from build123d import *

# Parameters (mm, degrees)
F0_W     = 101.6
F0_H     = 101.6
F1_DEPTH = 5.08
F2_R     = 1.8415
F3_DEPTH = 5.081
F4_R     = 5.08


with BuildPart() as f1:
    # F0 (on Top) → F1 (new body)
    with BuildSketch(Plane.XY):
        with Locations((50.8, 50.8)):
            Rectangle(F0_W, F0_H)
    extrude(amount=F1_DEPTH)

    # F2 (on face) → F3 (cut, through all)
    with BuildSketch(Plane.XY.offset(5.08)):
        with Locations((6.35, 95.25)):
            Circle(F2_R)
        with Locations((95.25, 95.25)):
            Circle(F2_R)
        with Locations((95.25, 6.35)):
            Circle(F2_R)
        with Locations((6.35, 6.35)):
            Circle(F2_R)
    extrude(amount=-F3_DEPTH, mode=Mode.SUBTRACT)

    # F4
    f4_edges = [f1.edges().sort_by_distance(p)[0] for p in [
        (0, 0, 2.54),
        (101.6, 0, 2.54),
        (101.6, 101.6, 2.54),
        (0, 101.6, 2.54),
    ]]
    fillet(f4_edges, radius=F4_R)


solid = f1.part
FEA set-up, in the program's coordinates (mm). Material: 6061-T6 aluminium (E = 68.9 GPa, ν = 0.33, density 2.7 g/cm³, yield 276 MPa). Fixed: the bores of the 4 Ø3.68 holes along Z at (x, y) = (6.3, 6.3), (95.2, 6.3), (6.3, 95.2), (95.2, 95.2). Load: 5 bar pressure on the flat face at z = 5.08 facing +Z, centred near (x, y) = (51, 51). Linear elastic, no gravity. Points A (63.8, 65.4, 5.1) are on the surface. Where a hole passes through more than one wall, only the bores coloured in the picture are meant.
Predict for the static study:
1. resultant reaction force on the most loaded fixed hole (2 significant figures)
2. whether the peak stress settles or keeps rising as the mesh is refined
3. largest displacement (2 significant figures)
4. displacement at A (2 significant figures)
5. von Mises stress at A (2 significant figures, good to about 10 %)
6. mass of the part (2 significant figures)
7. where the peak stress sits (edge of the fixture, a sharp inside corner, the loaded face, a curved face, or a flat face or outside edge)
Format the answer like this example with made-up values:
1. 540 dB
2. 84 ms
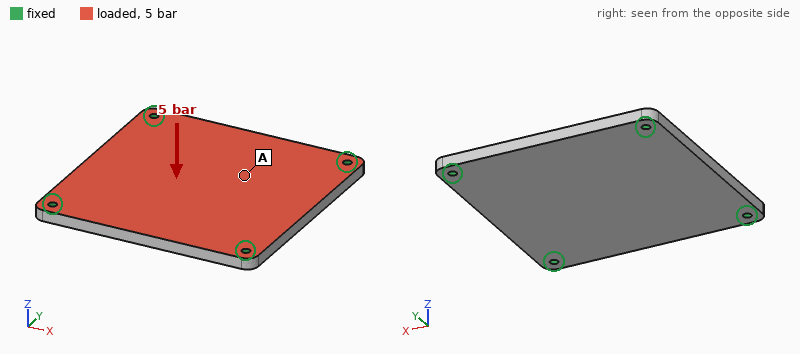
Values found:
1. 1.3 kN
2. keeps rising
3. 0.33 mm
4. 0.29 mm
5. 48 MPa
6. 140 g
7. edge of the fixture
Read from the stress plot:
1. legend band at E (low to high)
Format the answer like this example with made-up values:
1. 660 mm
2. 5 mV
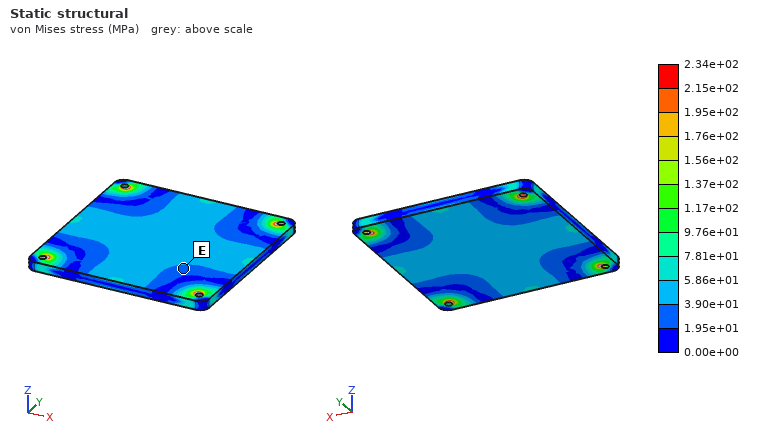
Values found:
1. 1.95e+01 to 3.90e+01 MPa
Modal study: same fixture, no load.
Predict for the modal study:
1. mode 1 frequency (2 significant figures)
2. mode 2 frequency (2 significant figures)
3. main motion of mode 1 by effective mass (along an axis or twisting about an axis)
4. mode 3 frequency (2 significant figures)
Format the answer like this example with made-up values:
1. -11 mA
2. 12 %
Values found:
1. 2000 Hz
2. 3500 Hz
3. along Z
4. 3500 Hz
